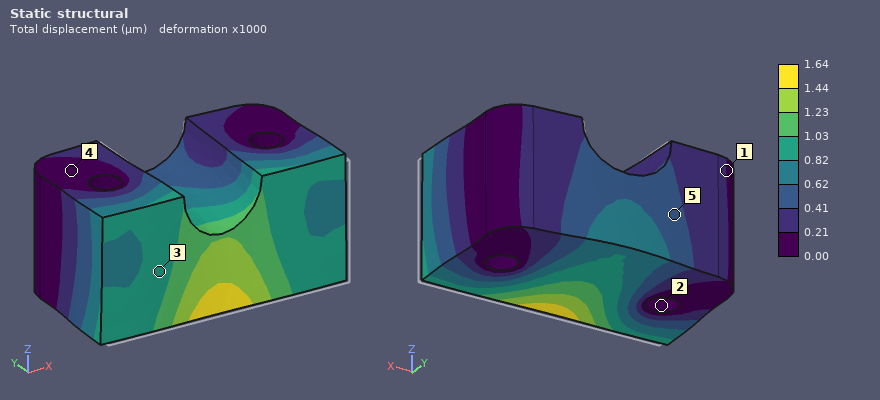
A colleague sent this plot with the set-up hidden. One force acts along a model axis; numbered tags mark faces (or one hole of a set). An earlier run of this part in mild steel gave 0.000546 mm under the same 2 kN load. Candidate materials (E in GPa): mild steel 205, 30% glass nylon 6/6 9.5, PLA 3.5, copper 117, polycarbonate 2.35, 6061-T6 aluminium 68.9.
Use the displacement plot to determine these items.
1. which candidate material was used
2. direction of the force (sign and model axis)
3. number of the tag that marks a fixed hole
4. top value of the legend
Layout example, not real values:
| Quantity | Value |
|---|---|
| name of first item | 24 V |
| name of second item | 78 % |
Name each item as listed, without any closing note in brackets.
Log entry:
| Quantity | Value |
|---|---|
| which candidate material was used | 6061-T6 aluminium |
| direction of the force | +Y |
| number of the tag that marks a fixed hole | 2 |
| top value of the legend | 1.64 µm |
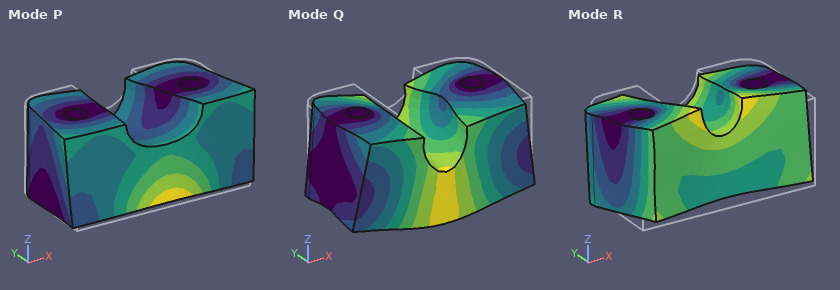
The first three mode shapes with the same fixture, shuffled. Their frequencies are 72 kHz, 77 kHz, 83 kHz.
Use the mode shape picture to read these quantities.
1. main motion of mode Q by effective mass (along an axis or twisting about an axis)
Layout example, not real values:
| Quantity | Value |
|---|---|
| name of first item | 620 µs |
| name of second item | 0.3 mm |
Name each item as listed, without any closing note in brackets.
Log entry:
| Quantity | Value |
|---|---|
| main motion of mode Q by effective mass | along Z |
